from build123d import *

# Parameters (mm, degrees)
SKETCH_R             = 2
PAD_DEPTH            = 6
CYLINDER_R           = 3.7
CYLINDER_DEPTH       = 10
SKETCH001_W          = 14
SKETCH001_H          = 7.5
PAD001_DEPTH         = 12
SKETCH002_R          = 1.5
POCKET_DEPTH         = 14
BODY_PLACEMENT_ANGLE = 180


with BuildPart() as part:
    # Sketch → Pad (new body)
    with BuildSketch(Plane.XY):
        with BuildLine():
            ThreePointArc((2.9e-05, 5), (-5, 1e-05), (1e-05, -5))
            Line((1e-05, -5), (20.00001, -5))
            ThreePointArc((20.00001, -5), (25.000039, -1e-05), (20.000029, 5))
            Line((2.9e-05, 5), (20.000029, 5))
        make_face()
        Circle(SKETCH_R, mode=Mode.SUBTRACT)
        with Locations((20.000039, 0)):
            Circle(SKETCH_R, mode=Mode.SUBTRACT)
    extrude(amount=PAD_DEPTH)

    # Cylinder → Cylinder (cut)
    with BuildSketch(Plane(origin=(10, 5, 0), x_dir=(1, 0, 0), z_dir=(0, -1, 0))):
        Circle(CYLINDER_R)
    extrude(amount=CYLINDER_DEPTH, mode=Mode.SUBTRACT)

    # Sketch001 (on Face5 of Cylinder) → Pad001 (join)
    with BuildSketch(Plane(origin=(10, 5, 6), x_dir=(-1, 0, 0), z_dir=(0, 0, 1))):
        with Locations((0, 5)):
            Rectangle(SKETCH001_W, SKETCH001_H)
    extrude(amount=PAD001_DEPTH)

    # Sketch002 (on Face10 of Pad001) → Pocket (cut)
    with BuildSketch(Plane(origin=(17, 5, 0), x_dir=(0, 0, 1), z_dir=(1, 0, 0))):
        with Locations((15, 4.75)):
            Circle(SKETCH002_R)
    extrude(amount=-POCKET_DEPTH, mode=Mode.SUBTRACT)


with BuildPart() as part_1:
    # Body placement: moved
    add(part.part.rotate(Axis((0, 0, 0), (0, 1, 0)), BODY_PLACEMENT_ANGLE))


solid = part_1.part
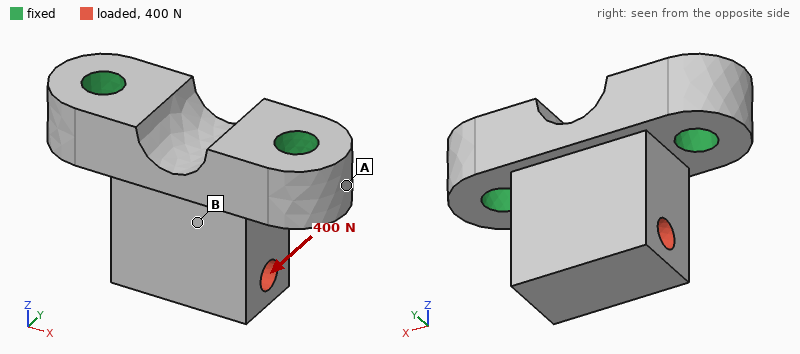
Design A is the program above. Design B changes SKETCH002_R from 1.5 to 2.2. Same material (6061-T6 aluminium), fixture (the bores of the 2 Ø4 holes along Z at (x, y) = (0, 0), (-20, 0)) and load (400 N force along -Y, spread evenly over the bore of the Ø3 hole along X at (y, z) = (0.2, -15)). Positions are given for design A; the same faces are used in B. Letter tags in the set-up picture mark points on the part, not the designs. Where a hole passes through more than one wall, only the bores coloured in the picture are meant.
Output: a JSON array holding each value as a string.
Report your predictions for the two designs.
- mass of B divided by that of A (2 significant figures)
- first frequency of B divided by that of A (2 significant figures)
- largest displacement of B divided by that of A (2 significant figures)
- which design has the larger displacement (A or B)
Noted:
["0.95", "1.1", "1.1", "B"]
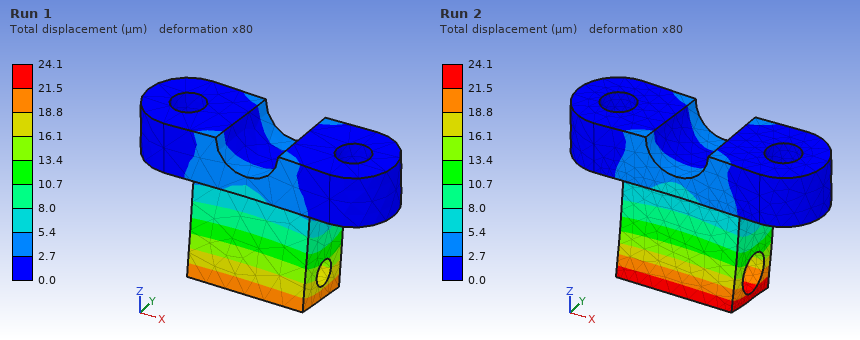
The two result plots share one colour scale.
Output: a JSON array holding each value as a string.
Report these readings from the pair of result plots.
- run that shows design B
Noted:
["Run 2"]
